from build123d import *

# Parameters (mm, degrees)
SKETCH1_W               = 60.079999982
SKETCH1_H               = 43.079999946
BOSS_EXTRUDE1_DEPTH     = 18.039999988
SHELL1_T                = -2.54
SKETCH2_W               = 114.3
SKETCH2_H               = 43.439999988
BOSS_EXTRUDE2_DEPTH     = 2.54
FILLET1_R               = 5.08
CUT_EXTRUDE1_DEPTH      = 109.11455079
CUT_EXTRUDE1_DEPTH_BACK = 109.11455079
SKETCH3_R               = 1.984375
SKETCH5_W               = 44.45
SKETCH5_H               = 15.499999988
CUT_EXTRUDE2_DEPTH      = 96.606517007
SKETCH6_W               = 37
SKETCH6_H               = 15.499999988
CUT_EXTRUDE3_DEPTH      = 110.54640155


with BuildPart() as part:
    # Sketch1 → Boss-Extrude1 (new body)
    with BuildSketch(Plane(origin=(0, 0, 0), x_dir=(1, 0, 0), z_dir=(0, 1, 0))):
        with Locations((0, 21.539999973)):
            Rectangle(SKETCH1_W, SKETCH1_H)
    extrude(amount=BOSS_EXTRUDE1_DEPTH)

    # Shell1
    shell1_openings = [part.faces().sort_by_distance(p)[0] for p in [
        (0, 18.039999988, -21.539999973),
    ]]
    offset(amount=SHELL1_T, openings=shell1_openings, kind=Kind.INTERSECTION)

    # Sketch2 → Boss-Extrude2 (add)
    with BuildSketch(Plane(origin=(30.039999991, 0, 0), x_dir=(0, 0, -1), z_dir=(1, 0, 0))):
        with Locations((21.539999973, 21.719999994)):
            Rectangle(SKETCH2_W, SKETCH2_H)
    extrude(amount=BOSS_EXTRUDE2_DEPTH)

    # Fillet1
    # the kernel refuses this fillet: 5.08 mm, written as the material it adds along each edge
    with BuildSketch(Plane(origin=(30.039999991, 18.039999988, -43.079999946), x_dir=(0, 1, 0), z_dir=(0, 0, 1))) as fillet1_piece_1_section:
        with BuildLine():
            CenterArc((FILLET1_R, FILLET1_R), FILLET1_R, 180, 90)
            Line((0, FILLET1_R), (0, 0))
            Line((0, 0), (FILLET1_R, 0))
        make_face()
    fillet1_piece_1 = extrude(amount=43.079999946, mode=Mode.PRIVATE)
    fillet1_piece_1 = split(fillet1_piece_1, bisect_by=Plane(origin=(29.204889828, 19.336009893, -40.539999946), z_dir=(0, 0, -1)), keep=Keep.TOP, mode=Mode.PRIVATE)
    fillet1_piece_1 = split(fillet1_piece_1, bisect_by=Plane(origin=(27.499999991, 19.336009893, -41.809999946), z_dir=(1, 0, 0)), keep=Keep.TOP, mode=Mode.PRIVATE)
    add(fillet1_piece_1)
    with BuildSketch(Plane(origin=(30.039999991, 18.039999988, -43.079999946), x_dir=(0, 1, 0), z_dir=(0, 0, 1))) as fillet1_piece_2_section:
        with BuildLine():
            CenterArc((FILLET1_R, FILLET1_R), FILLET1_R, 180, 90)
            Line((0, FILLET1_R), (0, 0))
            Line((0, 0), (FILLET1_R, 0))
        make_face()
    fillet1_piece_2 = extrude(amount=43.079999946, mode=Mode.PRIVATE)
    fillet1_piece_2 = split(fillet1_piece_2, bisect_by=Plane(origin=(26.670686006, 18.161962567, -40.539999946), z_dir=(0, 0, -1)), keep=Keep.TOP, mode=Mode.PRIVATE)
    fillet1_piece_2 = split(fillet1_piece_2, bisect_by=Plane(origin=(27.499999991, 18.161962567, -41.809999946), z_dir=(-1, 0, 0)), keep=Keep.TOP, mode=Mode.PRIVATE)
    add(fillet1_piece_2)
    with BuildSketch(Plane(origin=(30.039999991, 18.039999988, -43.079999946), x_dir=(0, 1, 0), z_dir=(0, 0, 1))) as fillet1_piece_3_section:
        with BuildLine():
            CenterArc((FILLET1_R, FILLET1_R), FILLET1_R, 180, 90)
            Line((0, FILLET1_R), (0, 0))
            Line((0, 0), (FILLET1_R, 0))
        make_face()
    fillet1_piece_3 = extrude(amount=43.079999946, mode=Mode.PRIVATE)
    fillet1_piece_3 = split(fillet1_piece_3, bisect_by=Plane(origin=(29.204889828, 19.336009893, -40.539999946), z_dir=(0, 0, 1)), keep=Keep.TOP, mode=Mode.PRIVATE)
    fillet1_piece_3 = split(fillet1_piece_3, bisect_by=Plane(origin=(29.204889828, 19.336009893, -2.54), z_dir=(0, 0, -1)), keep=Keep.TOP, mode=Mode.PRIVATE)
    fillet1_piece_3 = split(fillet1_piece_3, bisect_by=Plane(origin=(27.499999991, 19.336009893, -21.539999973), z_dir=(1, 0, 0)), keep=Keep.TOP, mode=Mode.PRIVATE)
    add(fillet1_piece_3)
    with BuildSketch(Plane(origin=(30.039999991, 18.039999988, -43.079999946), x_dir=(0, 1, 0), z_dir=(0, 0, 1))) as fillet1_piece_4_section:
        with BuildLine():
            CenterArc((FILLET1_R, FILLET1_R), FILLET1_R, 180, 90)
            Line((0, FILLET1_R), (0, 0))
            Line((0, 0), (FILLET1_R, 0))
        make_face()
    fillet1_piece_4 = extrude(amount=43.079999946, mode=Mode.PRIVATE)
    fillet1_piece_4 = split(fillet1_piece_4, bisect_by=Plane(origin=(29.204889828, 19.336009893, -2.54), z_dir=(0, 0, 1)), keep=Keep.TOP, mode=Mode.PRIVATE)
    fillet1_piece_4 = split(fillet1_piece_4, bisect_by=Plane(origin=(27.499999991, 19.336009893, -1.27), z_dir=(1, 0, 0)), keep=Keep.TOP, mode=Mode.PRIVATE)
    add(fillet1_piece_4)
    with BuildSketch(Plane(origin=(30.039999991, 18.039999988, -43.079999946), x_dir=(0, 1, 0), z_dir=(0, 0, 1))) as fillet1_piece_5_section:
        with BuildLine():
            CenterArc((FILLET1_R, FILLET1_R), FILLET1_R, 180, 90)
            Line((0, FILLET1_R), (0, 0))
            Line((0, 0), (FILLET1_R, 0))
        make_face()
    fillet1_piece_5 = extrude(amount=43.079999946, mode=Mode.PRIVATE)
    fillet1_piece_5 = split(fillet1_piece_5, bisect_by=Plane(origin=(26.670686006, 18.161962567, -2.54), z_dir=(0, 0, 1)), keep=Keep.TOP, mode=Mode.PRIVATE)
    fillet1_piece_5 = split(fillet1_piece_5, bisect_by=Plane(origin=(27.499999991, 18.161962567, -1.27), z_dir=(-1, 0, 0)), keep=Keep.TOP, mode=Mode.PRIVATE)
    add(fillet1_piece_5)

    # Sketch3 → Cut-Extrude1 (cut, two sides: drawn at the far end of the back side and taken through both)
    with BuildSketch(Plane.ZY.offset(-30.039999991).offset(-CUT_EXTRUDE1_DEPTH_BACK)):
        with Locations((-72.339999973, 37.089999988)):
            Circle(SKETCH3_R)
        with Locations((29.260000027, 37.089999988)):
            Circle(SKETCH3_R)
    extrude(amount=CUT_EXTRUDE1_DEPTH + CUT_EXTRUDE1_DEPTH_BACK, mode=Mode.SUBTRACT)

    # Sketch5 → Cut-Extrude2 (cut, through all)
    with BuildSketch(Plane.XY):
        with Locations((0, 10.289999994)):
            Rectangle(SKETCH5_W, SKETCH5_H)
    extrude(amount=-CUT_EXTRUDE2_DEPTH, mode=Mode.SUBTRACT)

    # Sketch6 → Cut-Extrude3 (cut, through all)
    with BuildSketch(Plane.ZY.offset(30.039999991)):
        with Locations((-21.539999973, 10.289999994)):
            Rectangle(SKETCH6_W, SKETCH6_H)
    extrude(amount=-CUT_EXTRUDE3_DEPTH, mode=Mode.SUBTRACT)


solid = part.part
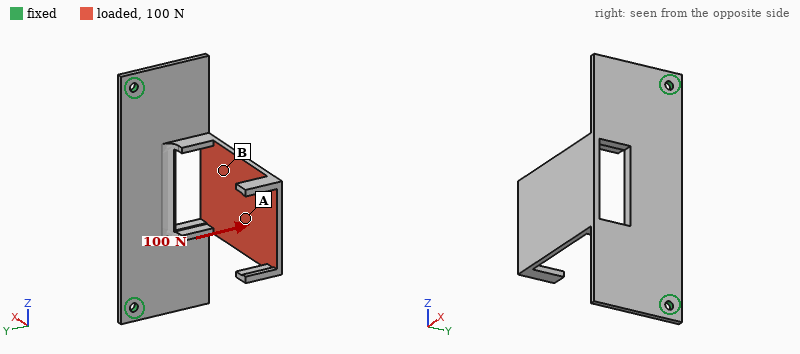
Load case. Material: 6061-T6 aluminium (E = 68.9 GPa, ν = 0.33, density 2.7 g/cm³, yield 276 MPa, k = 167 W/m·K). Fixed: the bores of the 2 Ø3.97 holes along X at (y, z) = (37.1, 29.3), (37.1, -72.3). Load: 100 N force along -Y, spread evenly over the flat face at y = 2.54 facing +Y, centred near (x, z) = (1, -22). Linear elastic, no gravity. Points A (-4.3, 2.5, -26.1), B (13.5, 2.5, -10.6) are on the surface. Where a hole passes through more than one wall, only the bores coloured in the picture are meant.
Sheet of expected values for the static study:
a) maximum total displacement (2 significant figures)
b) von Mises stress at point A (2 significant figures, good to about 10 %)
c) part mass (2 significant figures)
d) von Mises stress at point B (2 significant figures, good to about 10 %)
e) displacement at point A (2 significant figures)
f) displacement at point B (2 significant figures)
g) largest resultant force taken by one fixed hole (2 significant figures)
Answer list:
1.6 mm
15 MPa
52 g
34 MPa
0.86 mm
0.49 mm
69 N
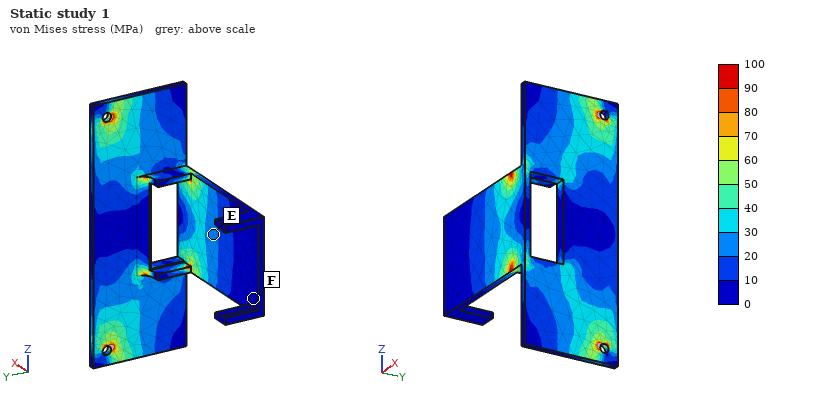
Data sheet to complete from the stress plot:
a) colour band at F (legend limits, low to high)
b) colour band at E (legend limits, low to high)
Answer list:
0 to 10 MPa
20 to 30 MPa
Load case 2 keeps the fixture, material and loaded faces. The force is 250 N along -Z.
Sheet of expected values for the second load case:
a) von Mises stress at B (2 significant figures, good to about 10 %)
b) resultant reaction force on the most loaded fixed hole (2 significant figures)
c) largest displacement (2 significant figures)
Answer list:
22 MPa
170 N
0.82 mm
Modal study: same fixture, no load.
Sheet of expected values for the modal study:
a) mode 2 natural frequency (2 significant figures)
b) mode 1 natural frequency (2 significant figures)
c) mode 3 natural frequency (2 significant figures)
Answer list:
670 Hz
290 Hz
680 Hz
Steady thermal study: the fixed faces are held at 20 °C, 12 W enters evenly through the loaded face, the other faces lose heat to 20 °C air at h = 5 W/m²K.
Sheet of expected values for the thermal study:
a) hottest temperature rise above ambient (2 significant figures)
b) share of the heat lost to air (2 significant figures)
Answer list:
45 K
11 %
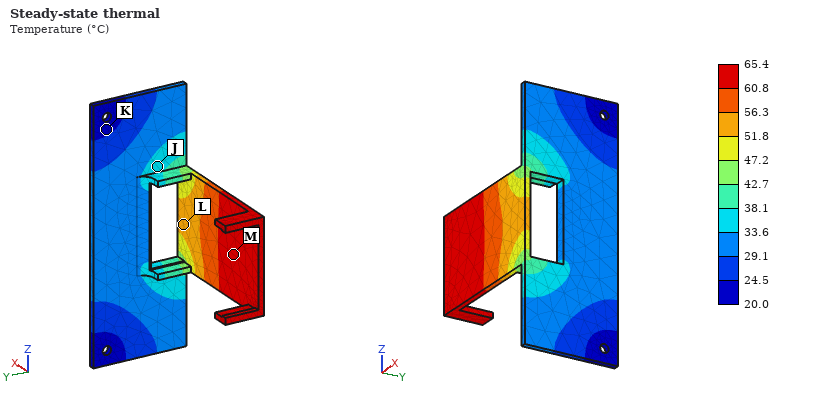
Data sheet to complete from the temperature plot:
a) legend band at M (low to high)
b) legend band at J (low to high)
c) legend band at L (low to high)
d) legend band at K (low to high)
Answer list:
60.8 to 65.4 °C
33.6 to 38.1 °C
51.8 to 56.3 °C
20.0 to 24.5 °C
